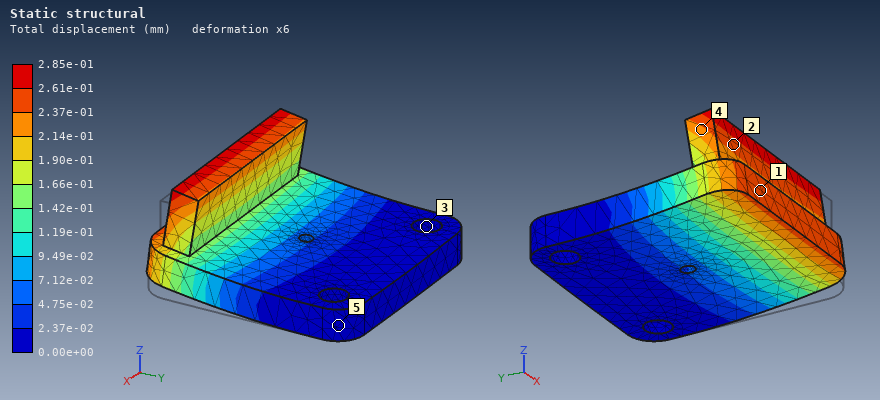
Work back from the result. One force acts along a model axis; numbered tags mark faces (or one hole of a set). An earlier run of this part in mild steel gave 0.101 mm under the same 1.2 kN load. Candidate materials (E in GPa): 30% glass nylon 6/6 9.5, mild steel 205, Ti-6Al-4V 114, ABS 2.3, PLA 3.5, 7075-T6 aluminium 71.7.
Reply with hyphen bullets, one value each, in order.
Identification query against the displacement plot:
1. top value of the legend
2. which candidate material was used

- 2.85e-01 mm
- 7075-T6 aluminium
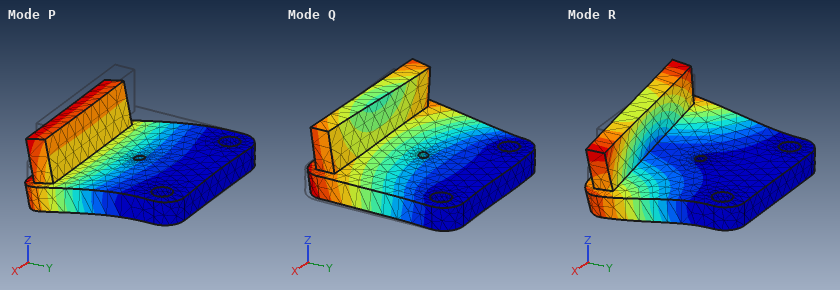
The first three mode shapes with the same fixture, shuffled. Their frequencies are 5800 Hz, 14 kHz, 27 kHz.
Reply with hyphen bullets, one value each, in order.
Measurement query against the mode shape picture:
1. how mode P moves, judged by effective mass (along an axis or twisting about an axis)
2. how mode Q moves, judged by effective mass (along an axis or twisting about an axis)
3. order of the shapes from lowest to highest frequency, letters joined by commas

- along Z
- along X
- P, R, Q
